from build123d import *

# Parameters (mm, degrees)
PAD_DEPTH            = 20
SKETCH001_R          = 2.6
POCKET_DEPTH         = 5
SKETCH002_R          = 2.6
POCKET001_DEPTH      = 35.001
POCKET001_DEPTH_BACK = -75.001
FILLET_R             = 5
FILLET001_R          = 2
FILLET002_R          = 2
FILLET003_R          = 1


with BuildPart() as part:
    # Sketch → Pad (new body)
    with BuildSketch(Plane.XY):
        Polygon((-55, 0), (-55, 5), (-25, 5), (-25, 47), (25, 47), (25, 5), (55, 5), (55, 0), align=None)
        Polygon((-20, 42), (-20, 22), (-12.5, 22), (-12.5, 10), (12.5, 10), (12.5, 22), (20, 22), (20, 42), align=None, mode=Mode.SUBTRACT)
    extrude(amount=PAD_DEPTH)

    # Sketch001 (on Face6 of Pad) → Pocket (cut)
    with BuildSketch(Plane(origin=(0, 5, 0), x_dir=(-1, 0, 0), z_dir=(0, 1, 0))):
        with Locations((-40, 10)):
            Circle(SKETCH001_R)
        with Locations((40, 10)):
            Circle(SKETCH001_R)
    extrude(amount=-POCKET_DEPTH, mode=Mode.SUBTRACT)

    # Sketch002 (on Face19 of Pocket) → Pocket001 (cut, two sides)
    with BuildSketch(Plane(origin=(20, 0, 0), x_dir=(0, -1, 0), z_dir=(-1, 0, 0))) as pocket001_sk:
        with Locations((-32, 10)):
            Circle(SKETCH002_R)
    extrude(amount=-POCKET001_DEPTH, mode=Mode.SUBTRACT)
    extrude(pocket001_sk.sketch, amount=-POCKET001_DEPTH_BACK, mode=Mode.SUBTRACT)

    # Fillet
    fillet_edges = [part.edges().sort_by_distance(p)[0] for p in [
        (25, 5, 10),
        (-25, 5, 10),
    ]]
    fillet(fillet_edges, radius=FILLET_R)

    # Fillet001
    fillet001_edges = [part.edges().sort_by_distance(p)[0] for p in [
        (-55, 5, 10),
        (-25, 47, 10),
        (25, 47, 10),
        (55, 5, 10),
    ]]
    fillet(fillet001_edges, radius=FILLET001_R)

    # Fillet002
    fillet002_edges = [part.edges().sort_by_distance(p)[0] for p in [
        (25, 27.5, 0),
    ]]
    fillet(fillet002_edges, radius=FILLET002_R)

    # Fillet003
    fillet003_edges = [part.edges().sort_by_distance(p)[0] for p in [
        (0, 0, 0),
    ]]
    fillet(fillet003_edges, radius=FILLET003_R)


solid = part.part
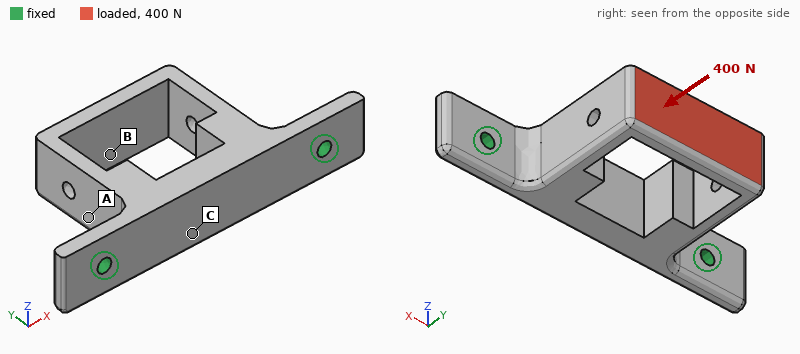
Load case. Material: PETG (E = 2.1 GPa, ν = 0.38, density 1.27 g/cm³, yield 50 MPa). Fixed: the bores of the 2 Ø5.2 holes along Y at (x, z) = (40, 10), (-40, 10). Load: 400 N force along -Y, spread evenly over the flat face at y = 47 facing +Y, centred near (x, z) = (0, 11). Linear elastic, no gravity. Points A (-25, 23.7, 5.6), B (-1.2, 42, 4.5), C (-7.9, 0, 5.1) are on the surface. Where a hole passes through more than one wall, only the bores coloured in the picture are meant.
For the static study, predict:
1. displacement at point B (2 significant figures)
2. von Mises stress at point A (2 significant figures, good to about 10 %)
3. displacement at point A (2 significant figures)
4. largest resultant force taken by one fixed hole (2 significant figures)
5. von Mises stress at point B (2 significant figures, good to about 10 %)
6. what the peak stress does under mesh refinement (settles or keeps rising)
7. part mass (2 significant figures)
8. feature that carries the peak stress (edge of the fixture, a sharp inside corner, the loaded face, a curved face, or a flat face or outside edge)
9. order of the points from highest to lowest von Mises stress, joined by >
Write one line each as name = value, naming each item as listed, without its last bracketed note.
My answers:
displacement at point B = 0.57 mm
von Mises stress at point A = 3.9 MPa
displacement at point A = 0.20 mm
largest resultant force taken by one fixed hole = 230 N
von Mises stress at point B = 11 MPa
what the peak stress does under mesh refinement = keeps rising
part mass = 39 g
feature that carries the peak stress = edge of the fixture
order of the points from highest to lowest von Mises stress, joined by > = B > A > C
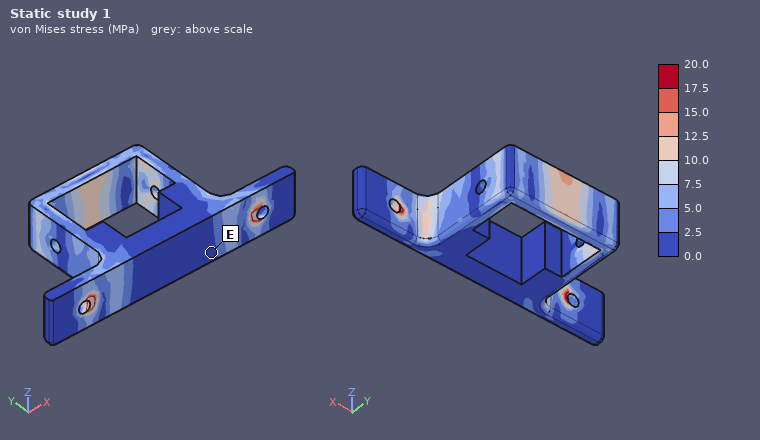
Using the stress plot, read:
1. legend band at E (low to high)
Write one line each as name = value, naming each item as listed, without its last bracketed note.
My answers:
legend band at E = 0.0 to 2.5 MPa
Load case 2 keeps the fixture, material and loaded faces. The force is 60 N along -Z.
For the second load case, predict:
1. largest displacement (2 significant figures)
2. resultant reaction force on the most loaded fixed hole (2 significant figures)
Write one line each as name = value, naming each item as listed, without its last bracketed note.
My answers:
largest displacement = 1.3 mm
resultant reaction force on the most loaded fixed hole = 30 N
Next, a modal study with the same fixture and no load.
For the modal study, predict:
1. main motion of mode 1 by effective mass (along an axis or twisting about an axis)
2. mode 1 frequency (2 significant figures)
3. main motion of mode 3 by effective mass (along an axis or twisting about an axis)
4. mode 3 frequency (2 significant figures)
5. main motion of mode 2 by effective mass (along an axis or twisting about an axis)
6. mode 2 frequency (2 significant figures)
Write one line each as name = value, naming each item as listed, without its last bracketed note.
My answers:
main motion of mode 1 by effective mass = along Z
mode 1 frequency = 370 Hz
main motion of mode 3 by effective mass = along Y
mode 3 frequency = 1100 Hz
main motion of mode 2 by effective mass = along X
mode 2 frequency = 920 Hz
